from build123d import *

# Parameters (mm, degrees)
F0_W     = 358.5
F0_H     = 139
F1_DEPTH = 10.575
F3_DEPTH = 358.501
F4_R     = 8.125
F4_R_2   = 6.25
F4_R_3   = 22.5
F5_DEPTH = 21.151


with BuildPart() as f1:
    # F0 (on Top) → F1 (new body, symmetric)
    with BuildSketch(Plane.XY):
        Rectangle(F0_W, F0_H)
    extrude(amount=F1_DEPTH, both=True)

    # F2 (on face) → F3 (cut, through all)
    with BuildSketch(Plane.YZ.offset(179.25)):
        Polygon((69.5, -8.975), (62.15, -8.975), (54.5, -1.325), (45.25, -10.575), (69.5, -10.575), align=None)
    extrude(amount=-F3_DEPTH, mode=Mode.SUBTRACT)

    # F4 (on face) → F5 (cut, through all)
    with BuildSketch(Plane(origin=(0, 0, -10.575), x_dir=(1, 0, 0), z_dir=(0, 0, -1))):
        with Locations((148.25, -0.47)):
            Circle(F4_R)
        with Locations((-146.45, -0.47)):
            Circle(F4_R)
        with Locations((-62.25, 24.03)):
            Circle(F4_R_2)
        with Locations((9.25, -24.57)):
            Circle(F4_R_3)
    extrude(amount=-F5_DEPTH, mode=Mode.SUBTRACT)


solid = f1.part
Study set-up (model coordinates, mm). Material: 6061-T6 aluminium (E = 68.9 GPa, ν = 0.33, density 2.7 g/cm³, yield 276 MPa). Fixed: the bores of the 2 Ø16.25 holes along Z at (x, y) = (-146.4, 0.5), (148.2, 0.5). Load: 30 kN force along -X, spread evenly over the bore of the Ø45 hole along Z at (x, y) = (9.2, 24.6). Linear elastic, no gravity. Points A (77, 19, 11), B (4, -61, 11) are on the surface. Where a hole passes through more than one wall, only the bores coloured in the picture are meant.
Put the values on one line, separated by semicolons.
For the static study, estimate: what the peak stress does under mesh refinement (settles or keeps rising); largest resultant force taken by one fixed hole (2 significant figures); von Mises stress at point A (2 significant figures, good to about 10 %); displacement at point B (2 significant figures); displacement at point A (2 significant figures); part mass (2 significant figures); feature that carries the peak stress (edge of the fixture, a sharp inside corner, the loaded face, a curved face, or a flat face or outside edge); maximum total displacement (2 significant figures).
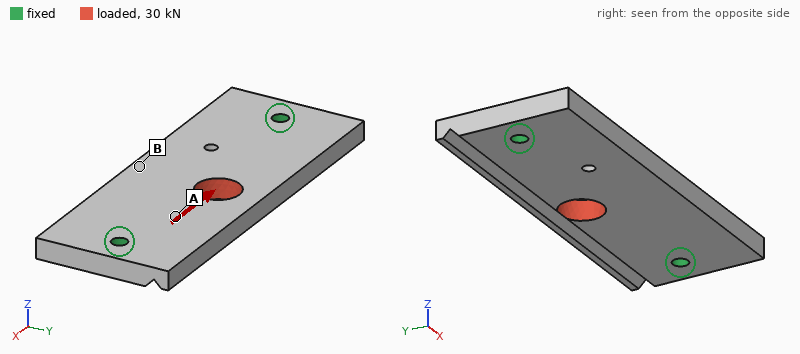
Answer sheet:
keeps rising; 16 kN; 9.3 MPa; 9.0 µm; 12 µm; 2.6 kg; edge of the fixture; 25 µm
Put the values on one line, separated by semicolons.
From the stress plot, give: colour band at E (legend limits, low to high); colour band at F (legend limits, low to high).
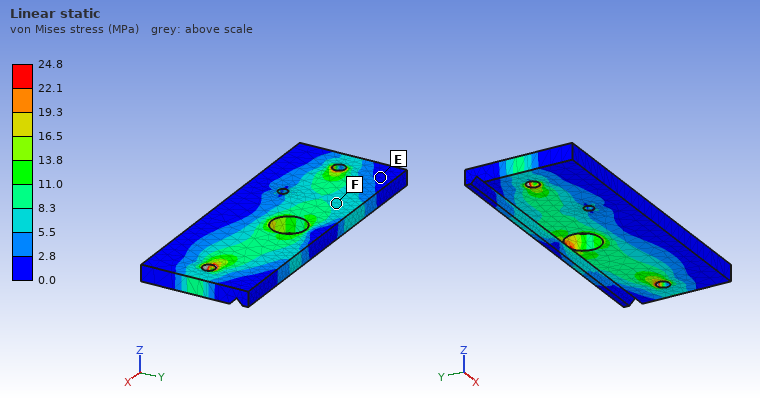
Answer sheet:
0.0 to 2.8 MPa; 5.5 to 8.3 MPa
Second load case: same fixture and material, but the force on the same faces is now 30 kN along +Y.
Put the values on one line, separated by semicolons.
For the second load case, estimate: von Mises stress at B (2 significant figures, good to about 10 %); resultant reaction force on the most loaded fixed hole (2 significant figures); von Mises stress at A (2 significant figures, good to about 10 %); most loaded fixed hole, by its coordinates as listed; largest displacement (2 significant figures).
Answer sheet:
27 MPa; 16 kN; 13 MPa; (148.2, 0.5); 0.10 mm
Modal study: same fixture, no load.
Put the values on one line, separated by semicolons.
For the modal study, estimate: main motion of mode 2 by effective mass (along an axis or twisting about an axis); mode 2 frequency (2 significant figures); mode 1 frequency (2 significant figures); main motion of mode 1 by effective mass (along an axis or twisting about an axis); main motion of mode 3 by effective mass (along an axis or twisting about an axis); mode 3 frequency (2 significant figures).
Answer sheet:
twisting about X; 1400 Hz; 1100 Hz; along Z; twisting about Y; 2600 Hz
